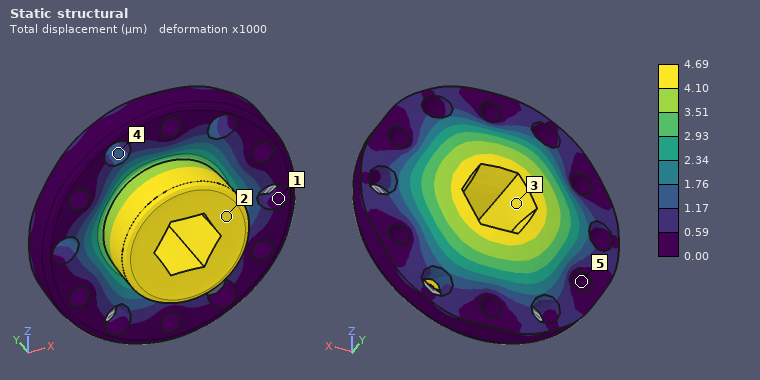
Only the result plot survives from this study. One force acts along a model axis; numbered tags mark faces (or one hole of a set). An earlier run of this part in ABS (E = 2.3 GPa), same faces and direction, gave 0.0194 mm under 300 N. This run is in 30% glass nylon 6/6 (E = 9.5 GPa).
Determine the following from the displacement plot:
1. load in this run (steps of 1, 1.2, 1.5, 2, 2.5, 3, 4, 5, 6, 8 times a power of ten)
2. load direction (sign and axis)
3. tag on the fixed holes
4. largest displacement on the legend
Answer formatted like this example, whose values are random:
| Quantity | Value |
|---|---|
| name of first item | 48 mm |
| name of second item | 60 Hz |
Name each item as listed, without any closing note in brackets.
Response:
| Quantity | Value |
|---|---|
| load in this run | 300 N |
| load direction | +Y |
| tag on the fixed holes | 5 |
| largest displacement on the legend | 4.69 µm |
